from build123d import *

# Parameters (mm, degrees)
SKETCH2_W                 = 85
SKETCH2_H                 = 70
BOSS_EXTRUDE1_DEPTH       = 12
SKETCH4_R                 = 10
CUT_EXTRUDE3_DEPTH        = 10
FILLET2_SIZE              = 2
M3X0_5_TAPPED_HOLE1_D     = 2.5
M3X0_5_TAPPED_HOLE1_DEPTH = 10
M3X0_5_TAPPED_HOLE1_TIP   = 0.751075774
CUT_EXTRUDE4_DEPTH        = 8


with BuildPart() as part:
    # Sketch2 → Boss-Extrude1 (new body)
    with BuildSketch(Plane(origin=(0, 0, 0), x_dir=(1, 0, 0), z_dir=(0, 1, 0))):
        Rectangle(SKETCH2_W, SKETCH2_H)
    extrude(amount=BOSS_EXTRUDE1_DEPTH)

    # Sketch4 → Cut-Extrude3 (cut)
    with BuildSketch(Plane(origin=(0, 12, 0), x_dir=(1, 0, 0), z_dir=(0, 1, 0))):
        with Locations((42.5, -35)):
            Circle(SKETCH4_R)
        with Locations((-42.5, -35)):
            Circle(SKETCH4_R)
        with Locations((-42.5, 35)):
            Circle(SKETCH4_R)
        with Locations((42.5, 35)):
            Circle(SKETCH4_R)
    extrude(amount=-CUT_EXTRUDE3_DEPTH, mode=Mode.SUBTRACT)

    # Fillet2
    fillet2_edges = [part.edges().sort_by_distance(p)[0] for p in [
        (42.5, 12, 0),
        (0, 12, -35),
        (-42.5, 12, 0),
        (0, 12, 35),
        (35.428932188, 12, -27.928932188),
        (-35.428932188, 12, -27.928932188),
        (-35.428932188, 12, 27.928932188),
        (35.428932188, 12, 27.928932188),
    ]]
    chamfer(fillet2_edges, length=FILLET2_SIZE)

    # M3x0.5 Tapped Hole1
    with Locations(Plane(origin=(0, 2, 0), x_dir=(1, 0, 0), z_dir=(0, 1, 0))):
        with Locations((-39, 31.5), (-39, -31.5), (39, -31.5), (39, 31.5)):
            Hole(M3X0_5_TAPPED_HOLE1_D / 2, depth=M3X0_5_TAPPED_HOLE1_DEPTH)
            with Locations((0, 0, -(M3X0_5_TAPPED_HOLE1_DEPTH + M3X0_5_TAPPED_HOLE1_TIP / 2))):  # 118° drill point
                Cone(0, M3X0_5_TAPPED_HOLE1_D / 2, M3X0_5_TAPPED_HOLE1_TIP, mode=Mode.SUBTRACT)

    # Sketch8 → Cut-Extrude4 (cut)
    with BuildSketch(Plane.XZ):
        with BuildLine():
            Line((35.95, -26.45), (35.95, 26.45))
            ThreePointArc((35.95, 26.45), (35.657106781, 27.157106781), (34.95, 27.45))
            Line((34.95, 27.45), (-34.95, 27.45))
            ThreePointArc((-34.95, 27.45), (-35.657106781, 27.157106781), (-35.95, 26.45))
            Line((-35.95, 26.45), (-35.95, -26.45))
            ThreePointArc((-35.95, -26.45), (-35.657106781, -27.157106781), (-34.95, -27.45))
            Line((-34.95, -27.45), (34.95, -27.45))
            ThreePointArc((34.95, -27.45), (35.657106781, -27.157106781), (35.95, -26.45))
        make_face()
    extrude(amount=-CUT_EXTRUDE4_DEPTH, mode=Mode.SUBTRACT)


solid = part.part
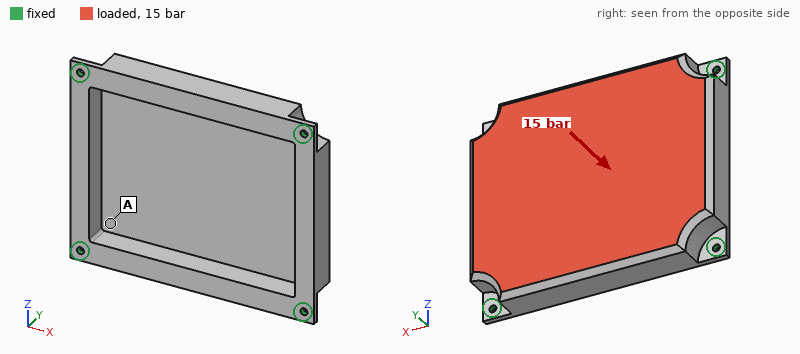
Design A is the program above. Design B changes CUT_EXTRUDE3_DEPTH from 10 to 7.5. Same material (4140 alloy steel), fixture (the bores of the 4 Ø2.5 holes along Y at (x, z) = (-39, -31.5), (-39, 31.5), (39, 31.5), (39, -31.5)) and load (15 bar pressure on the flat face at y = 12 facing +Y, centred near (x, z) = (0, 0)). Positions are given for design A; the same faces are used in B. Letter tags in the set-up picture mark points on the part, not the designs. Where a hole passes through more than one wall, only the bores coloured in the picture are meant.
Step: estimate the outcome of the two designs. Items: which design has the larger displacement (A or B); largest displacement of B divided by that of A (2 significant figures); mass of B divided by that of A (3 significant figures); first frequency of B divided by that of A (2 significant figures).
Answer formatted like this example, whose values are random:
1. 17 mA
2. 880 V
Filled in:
1. A
2. 0.79
3. 1.02
4. 1.2
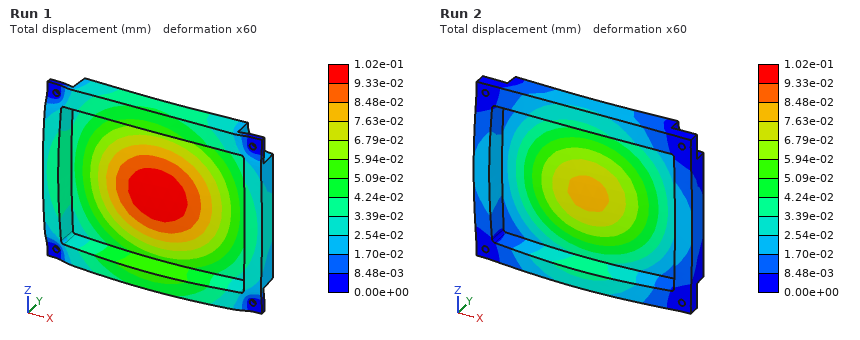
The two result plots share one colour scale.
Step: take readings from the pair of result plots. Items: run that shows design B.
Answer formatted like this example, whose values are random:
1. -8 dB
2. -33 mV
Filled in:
1. Run 2
